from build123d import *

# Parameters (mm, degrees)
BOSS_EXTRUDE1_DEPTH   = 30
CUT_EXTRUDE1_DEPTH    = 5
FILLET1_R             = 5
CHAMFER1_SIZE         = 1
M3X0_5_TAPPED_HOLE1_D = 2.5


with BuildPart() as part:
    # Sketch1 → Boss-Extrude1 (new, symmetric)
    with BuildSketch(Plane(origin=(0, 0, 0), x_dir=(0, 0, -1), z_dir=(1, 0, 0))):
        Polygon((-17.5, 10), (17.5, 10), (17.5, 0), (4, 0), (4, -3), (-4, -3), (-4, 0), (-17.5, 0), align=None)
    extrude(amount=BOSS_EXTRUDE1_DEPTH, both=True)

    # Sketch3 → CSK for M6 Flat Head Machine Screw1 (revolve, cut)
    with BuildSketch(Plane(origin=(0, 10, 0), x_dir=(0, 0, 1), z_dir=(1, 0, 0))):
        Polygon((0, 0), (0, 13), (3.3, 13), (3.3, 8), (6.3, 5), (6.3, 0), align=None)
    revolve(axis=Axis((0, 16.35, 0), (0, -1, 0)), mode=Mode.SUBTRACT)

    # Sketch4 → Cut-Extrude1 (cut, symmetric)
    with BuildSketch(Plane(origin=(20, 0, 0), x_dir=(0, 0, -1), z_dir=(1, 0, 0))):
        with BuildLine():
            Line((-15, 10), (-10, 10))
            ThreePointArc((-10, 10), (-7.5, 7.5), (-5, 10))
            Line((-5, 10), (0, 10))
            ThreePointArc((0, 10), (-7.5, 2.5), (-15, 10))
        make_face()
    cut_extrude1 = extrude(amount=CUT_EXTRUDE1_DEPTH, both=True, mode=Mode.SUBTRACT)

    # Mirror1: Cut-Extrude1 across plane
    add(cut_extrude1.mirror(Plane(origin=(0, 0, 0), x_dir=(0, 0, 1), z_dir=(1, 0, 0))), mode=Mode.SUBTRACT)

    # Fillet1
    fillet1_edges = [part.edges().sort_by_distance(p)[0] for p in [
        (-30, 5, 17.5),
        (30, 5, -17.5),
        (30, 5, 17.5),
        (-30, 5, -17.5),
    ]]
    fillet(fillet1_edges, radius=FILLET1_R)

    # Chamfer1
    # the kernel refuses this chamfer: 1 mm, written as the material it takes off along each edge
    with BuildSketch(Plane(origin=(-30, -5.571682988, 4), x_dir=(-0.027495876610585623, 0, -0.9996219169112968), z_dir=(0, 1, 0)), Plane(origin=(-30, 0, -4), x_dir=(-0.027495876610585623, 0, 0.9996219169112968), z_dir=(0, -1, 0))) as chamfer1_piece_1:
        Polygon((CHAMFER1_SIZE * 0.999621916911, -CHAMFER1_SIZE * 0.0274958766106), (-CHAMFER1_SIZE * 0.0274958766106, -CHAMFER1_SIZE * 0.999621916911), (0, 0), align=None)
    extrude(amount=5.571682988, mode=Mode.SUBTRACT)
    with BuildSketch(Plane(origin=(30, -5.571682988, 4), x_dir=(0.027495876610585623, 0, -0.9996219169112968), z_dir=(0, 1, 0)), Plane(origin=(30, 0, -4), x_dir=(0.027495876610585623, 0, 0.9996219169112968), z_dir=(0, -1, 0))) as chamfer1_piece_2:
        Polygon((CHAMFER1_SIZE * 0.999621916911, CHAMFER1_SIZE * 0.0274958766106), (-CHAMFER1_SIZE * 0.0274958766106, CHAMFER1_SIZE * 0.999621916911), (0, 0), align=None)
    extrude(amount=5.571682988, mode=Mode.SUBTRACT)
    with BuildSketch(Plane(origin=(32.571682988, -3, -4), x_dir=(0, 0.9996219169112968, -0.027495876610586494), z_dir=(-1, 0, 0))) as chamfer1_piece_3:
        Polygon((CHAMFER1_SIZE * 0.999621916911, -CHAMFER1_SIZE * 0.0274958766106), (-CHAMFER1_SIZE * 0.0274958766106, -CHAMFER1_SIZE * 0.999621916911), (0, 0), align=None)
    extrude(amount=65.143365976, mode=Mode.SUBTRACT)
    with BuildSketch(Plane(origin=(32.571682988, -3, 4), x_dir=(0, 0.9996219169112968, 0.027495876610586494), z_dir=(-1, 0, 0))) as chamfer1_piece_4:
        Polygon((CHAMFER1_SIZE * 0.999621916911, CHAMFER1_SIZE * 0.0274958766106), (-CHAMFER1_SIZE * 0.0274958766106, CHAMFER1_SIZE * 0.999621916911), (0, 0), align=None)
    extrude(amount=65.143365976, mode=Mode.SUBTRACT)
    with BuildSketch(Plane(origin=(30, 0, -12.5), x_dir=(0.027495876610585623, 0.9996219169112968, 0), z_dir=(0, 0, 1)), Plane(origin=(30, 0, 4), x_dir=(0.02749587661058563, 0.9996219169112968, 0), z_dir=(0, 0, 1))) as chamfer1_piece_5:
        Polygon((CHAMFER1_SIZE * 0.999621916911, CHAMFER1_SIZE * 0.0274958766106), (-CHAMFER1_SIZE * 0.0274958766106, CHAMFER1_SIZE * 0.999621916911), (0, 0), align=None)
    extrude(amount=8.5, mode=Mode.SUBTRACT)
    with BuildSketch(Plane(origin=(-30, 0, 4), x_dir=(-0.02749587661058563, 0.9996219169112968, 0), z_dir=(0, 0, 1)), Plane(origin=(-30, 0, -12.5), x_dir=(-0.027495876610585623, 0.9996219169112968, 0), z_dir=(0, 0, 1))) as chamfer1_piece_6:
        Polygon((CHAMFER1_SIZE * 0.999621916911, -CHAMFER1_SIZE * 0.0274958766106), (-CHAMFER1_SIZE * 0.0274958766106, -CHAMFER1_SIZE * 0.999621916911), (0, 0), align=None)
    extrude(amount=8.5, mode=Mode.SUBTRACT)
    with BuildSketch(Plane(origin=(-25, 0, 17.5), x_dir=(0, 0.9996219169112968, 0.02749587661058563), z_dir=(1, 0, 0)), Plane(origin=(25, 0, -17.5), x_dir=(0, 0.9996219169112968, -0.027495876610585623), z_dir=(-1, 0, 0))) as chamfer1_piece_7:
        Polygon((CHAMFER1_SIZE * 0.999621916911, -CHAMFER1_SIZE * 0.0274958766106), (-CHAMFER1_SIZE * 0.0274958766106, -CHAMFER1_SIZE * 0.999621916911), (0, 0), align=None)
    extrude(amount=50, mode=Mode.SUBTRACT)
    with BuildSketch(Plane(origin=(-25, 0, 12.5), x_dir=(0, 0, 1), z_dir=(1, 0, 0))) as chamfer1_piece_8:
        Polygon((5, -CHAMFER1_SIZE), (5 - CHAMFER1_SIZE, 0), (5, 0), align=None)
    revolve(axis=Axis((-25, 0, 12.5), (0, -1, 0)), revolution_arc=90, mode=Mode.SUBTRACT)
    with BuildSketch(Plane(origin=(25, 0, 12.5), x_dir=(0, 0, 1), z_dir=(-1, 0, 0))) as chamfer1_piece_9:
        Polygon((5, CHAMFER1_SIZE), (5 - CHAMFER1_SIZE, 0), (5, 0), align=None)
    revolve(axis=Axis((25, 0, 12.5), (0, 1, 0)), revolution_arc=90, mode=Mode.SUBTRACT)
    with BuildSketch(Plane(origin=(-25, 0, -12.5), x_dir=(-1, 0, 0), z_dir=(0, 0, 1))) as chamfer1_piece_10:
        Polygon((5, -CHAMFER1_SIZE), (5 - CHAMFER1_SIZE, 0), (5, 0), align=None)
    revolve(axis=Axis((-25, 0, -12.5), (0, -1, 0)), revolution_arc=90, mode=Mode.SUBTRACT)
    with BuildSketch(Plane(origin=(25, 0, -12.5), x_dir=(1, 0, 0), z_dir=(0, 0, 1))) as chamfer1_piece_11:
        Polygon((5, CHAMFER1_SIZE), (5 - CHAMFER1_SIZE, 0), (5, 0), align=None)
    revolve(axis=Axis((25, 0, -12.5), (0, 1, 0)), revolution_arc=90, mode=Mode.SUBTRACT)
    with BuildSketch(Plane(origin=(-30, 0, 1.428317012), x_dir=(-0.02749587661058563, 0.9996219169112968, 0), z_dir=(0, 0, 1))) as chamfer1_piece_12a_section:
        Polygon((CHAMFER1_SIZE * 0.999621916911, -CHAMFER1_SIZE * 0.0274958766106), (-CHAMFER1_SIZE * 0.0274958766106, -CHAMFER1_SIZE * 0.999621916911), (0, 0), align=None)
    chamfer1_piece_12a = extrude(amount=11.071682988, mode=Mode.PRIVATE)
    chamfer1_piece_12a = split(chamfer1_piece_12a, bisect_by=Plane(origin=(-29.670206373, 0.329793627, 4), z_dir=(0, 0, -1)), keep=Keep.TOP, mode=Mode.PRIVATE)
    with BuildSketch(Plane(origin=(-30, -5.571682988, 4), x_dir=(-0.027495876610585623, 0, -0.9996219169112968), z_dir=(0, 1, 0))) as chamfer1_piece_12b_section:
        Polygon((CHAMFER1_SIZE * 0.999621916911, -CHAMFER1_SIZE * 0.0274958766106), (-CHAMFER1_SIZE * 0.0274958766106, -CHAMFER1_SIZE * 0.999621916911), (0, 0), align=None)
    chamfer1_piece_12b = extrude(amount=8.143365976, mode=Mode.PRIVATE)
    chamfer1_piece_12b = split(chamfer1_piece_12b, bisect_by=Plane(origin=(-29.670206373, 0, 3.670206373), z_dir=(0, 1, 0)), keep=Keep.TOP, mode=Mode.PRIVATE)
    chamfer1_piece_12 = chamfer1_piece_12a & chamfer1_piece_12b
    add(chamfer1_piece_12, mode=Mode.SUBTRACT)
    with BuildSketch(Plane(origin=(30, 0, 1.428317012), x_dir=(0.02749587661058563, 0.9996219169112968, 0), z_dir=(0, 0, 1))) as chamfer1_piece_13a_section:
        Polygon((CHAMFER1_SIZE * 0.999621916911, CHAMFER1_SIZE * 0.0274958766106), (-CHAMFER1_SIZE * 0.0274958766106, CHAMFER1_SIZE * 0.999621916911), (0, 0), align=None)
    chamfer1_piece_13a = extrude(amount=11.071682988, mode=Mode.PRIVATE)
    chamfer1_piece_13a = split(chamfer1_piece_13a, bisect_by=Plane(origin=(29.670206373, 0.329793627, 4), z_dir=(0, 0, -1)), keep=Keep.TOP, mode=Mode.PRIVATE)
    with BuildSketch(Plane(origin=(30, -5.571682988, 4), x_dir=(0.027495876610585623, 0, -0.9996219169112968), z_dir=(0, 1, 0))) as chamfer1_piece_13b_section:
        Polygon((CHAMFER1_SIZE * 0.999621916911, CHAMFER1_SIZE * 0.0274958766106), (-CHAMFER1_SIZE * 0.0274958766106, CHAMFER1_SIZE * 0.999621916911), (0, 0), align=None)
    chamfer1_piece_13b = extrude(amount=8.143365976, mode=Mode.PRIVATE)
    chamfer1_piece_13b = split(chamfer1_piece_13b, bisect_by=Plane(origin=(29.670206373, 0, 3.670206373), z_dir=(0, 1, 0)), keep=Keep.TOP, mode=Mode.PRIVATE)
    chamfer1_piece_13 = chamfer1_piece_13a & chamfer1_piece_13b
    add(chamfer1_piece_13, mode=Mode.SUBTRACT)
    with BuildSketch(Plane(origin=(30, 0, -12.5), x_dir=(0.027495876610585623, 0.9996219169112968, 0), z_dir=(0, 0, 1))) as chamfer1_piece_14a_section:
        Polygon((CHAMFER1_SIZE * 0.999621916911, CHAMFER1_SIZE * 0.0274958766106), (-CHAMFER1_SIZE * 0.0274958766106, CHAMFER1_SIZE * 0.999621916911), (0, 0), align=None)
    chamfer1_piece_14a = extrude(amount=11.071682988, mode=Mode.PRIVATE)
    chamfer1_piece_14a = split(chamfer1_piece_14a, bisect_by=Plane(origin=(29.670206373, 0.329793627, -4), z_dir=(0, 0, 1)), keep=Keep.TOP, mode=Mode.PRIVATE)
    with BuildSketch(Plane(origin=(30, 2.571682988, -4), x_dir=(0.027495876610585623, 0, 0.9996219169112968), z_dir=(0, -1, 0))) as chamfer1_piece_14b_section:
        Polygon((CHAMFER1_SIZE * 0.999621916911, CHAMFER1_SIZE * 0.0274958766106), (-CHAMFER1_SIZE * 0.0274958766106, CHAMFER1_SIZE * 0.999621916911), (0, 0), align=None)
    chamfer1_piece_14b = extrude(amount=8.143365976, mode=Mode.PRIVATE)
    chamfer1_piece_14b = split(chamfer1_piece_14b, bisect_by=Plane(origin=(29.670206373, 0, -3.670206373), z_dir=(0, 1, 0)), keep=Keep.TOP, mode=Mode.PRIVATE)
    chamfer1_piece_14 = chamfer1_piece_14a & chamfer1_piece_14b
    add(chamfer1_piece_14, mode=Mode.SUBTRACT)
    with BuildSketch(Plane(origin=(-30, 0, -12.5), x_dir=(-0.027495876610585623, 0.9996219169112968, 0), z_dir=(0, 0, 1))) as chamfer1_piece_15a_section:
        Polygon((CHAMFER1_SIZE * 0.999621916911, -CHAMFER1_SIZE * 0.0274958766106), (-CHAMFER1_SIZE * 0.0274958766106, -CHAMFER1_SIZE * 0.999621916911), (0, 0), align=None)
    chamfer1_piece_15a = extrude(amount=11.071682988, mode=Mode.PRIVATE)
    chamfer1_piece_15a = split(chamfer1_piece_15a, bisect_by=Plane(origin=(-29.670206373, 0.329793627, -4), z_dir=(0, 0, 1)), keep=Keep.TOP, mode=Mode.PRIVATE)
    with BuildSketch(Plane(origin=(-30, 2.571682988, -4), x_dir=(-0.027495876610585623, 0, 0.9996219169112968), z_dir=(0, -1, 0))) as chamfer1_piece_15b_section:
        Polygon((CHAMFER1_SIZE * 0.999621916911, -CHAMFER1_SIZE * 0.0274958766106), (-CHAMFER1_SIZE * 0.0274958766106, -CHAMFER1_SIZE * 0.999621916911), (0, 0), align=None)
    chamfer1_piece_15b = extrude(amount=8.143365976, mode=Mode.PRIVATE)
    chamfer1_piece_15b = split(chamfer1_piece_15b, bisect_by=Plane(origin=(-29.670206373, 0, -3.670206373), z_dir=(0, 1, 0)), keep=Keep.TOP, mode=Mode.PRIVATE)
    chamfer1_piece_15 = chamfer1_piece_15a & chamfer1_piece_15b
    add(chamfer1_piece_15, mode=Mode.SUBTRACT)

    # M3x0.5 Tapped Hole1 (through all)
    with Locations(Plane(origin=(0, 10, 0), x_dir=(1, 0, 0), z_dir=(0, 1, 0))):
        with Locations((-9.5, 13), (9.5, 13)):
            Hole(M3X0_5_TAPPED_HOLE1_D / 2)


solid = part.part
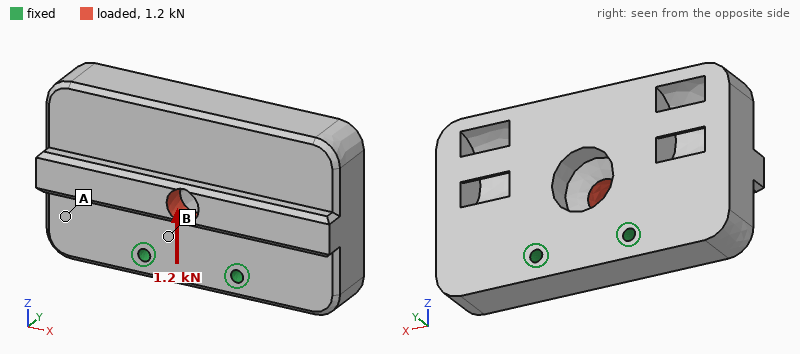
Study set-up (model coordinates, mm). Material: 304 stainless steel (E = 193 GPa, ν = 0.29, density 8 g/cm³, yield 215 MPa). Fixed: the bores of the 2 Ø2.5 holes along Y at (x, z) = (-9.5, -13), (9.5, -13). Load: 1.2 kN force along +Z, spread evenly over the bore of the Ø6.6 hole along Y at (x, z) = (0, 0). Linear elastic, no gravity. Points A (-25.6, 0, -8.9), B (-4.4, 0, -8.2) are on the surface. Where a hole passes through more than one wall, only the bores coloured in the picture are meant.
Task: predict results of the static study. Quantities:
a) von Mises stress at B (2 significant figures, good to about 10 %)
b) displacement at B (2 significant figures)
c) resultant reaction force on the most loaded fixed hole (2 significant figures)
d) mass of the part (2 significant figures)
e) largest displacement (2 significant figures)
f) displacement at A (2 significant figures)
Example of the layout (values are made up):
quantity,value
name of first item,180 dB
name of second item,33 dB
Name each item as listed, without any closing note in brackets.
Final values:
quantity,value
von Mises stress at B,15 MPa
displacement at B,0.82 µm
resultant reaction force on the most loaded fixed hole,610 N
mass of the part,160 g
largest displacement,4.8 µm
displacement at A,0.83 µm
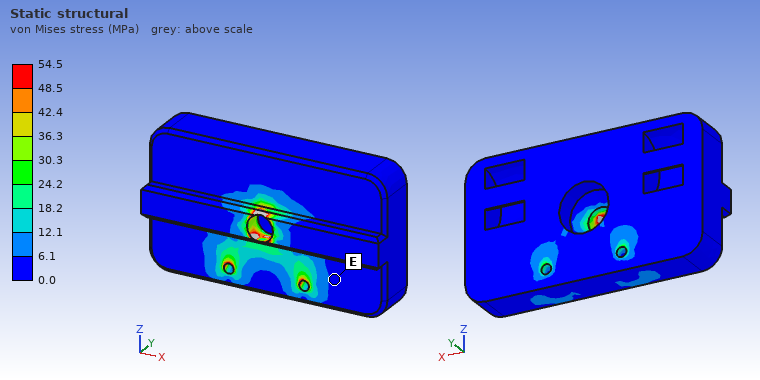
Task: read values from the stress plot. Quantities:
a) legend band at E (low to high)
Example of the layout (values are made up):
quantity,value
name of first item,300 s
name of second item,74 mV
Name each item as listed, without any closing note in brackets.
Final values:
quantity,value
legend band at E,0.0 to 6.1 MPa
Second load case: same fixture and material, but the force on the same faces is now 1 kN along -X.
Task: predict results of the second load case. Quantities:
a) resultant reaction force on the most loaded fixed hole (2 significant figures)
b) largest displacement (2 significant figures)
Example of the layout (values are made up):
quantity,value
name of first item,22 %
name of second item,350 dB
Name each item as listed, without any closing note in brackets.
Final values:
quantity,value
resultant reaction force on the most loaded fixed hole,810 N
largest displacement,3.0 µm
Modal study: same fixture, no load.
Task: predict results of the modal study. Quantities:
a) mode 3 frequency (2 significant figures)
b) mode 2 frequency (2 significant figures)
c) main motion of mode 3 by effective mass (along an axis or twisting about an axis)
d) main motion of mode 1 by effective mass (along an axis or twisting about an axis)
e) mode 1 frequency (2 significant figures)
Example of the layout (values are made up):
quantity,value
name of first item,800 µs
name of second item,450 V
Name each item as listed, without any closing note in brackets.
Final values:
quantity,value
mode 3 frequency,8400 Hz
mode 2 frequency,7300 Hz
main motion of mode 3 by effective mass,along X
main motion of mode 1 by effective mass,along Y
mode 1 frequency,5500 Hz
